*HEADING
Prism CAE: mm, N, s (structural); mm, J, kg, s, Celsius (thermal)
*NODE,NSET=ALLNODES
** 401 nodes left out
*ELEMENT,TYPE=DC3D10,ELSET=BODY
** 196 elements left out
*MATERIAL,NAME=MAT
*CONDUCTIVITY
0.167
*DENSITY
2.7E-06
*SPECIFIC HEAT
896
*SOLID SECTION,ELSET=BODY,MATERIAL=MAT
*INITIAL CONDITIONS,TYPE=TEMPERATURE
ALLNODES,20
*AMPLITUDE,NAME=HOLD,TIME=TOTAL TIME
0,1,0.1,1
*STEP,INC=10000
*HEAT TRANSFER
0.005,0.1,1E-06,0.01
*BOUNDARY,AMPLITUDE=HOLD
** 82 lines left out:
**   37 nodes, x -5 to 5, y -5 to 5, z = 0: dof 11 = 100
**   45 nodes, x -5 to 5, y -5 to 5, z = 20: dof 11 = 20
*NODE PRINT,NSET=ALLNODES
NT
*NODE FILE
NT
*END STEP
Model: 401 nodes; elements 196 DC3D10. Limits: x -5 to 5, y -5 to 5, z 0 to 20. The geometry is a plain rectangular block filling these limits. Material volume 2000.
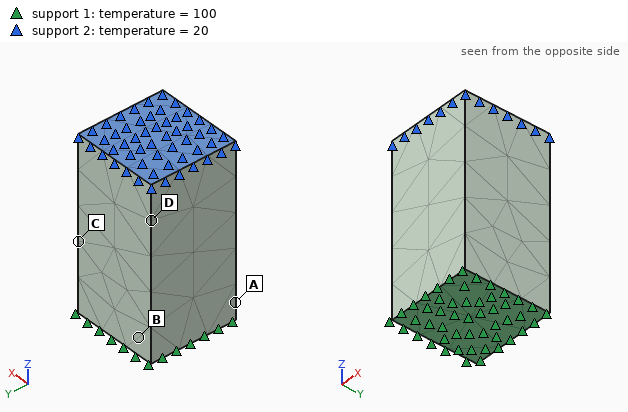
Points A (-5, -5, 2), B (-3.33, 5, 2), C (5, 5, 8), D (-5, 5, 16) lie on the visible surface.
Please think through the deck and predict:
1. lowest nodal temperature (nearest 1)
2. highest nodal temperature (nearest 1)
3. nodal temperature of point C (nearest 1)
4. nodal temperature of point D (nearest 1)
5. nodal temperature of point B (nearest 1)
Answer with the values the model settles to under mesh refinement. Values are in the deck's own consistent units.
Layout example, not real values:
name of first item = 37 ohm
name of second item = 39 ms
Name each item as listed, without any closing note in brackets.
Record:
lowest nodal temperature = 20
highest nodal temperature = 100
nodal temperature of point C = 23
nodal temperature of point D = 20
nodal temperature of point B = 67
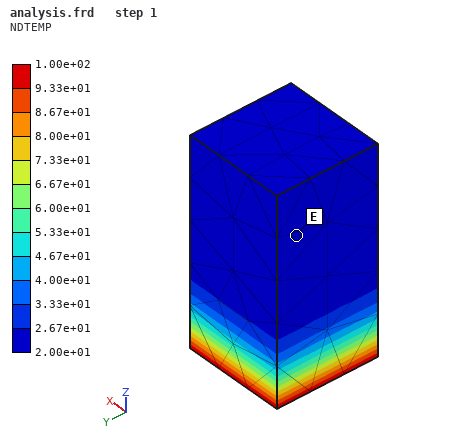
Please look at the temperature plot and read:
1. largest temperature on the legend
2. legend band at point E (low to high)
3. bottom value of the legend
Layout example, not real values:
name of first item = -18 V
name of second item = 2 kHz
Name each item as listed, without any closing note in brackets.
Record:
largest temperature on the legend = 1.00e+02
legend band at point E = 2.00e+01 to 2.67e+01
bottom value of the legend = 2.00e+01
